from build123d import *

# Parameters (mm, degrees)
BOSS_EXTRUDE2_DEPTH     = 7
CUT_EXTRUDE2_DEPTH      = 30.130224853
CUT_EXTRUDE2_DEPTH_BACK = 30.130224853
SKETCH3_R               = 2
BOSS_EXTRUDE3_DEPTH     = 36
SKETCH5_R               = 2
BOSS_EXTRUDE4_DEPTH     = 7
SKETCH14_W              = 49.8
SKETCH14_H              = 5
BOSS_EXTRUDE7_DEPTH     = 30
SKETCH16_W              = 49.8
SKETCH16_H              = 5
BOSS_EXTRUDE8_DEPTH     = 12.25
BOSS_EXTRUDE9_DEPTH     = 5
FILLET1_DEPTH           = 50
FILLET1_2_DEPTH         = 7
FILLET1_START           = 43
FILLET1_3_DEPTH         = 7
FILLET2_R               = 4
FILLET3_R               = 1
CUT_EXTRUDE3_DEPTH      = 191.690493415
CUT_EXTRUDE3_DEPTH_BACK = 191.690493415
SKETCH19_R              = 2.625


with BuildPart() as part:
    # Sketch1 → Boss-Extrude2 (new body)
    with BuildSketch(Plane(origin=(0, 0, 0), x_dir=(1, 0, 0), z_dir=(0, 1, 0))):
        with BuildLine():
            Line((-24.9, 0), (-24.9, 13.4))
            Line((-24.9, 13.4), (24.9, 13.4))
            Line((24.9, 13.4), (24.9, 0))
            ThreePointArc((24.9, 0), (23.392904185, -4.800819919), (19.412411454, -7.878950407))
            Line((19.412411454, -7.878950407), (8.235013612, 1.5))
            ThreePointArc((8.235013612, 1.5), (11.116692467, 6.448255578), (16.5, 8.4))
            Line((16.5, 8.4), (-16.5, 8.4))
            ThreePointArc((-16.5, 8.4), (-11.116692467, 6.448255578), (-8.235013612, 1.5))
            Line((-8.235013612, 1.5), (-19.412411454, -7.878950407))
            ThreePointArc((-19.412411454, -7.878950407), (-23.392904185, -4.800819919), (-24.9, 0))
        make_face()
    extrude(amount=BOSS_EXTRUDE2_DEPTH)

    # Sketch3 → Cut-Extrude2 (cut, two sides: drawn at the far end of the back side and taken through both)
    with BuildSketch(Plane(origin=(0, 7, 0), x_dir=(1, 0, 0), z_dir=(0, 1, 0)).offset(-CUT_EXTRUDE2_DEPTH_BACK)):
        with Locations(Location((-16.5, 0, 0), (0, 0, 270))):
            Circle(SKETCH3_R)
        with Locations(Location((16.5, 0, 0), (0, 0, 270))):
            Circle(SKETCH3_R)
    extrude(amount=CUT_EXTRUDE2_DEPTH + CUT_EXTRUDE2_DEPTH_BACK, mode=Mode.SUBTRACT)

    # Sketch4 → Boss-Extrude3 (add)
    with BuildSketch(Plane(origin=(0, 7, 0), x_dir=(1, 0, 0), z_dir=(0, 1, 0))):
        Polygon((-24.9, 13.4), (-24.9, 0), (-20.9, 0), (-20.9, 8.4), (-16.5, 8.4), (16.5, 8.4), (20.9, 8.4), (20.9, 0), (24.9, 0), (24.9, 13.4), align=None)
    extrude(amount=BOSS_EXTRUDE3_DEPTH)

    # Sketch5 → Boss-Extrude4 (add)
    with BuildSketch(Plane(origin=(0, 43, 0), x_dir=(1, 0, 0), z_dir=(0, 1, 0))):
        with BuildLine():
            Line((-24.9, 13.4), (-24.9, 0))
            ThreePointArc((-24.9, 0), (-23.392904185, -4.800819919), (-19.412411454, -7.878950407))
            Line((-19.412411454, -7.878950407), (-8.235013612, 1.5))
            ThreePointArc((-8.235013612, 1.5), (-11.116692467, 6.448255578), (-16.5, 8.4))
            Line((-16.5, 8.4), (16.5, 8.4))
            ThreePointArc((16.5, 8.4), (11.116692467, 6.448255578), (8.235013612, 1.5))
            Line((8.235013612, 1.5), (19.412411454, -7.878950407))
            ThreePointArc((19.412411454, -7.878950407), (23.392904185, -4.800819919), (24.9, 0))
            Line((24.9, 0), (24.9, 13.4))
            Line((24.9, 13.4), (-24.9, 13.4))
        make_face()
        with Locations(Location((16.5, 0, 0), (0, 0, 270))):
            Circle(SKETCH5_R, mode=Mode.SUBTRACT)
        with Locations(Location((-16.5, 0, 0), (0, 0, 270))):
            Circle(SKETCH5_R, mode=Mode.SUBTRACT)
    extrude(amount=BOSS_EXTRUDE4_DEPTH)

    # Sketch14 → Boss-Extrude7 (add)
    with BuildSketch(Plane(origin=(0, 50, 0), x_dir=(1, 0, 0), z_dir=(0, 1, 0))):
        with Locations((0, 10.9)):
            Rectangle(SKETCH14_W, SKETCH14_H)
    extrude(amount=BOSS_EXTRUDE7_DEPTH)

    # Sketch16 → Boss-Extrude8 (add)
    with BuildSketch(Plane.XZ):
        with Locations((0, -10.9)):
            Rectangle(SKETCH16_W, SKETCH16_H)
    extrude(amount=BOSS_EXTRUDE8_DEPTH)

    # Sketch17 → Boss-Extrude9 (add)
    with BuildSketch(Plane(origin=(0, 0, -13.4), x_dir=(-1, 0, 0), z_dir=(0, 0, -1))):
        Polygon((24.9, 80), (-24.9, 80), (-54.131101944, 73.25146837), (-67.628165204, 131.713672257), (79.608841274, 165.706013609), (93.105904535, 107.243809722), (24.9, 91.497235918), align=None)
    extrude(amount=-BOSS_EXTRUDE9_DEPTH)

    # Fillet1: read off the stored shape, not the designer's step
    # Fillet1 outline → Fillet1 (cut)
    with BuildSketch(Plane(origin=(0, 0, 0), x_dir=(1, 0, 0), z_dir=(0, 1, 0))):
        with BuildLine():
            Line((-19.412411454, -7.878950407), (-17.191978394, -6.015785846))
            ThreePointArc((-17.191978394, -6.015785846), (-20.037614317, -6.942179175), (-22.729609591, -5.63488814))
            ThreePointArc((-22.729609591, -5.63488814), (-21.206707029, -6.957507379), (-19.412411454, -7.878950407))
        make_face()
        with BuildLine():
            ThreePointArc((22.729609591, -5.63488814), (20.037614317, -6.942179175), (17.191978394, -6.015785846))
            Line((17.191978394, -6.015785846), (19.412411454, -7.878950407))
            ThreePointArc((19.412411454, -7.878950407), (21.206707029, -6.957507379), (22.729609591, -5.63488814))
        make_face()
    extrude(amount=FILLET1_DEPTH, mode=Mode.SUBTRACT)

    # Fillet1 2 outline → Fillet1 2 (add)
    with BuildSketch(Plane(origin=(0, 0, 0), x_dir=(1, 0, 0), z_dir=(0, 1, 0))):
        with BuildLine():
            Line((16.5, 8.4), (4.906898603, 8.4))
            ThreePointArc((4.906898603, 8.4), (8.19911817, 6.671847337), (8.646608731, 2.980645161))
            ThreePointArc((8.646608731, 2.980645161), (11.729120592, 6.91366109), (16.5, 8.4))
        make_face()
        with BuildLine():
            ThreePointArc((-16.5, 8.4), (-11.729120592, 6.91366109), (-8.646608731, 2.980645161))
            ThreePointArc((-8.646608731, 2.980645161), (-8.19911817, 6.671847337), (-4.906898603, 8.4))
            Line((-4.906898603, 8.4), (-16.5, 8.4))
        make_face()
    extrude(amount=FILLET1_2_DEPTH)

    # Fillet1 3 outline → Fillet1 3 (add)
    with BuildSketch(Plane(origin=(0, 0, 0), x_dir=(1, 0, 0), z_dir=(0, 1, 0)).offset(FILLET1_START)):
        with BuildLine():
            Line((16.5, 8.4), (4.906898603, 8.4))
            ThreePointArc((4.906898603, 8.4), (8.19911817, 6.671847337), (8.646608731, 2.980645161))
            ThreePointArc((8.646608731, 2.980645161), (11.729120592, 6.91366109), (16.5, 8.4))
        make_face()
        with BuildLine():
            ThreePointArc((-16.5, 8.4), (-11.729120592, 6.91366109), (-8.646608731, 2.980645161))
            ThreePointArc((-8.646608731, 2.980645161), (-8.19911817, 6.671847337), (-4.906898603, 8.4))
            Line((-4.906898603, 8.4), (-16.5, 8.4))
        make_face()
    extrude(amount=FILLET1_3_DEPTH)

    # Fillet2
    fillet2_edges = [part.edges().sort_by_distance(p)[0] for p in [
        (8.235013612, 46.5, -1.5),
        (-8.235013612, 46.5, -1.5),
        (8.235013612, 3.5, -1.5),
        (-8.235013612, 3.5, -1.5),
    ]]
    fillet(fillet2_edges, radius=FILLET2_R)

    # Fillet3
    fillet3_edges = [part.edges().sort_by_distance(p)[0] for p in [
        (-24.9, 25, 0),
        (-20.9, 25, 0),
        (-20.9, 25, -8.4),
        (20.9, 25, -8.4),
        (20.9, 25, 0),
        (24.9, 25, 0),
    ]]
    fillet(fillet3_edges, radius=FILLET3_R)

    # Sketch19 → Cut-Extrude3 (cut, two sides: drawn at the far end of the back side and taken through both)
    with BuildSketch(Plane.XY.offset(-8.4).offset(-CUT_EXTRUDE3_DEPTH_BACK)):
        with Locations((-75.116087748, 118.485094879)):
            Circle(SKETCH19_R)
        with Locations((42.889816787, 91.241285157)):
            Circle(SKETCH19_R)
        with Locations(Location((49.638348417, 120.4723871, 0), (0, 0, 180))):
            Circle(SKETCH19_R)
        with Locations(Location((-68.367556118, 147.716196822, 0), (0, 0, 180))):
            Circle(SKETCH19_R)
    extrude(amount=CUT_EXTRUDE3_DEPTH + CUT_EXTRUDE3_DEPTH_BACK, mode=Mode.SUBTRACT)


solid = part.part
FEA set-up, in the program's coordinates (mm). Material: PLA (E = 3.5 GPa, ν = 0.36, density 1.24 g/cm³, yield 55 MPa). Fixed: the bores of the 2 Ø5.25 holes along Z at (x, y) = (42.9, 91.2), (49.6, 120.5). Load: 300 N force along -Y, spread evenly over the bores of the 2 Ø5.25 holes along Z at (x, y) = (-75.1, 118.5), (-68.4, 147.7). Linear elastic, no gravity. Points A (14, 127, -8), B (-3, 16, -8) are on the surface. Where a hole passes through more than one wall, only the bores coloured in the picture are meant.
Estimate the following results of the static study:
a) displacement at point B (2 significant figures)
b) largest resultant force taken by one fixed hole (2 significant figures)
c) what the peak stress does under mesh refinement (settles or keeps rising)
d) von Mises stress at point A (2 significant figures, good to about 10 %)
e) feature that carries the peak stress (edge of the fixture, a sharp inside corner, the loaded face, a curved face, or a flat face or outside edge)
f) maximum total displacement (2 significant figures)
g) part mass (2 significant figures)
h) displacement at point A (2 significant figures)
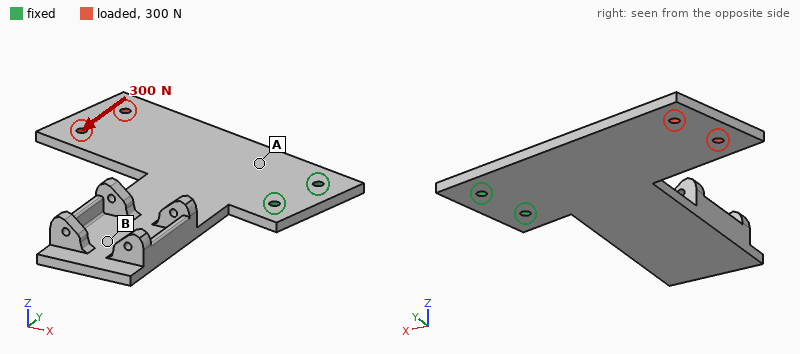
0.56 mm
1.1 kN
keeps rising
4.0 MPa
edge of the fixture
0.93 mm
96 g
0.17 mm
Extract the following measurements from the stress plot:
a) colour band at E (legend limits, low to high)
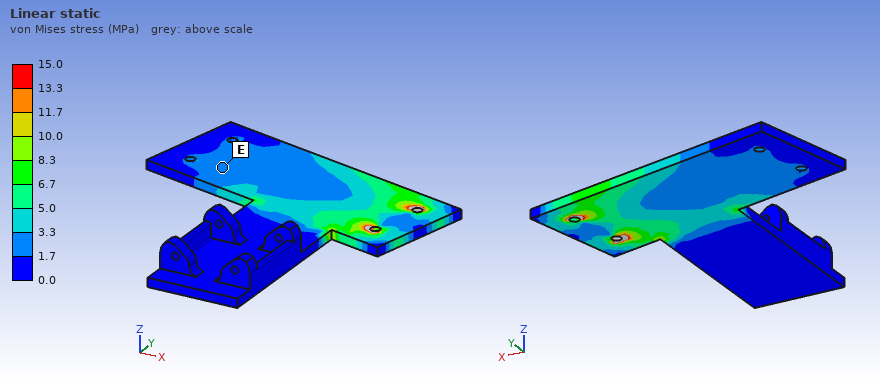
1.7 to 3.3 MPa
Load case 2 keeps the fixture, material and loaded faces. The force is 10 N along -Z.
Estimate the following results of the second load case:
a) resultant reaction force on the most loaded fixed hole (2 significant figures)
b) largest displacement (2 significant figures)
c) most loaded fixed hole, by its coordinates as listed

5.6 N
2.8 mm
(42.9, 91.2)
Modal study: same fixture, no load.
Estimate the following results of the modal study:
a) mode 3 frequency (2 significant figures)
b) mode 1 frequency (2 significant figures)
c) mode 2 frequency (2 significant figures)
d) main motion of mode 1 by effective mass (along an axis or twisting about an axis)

290 Hz
76 Hz
80 Hz
along Z
